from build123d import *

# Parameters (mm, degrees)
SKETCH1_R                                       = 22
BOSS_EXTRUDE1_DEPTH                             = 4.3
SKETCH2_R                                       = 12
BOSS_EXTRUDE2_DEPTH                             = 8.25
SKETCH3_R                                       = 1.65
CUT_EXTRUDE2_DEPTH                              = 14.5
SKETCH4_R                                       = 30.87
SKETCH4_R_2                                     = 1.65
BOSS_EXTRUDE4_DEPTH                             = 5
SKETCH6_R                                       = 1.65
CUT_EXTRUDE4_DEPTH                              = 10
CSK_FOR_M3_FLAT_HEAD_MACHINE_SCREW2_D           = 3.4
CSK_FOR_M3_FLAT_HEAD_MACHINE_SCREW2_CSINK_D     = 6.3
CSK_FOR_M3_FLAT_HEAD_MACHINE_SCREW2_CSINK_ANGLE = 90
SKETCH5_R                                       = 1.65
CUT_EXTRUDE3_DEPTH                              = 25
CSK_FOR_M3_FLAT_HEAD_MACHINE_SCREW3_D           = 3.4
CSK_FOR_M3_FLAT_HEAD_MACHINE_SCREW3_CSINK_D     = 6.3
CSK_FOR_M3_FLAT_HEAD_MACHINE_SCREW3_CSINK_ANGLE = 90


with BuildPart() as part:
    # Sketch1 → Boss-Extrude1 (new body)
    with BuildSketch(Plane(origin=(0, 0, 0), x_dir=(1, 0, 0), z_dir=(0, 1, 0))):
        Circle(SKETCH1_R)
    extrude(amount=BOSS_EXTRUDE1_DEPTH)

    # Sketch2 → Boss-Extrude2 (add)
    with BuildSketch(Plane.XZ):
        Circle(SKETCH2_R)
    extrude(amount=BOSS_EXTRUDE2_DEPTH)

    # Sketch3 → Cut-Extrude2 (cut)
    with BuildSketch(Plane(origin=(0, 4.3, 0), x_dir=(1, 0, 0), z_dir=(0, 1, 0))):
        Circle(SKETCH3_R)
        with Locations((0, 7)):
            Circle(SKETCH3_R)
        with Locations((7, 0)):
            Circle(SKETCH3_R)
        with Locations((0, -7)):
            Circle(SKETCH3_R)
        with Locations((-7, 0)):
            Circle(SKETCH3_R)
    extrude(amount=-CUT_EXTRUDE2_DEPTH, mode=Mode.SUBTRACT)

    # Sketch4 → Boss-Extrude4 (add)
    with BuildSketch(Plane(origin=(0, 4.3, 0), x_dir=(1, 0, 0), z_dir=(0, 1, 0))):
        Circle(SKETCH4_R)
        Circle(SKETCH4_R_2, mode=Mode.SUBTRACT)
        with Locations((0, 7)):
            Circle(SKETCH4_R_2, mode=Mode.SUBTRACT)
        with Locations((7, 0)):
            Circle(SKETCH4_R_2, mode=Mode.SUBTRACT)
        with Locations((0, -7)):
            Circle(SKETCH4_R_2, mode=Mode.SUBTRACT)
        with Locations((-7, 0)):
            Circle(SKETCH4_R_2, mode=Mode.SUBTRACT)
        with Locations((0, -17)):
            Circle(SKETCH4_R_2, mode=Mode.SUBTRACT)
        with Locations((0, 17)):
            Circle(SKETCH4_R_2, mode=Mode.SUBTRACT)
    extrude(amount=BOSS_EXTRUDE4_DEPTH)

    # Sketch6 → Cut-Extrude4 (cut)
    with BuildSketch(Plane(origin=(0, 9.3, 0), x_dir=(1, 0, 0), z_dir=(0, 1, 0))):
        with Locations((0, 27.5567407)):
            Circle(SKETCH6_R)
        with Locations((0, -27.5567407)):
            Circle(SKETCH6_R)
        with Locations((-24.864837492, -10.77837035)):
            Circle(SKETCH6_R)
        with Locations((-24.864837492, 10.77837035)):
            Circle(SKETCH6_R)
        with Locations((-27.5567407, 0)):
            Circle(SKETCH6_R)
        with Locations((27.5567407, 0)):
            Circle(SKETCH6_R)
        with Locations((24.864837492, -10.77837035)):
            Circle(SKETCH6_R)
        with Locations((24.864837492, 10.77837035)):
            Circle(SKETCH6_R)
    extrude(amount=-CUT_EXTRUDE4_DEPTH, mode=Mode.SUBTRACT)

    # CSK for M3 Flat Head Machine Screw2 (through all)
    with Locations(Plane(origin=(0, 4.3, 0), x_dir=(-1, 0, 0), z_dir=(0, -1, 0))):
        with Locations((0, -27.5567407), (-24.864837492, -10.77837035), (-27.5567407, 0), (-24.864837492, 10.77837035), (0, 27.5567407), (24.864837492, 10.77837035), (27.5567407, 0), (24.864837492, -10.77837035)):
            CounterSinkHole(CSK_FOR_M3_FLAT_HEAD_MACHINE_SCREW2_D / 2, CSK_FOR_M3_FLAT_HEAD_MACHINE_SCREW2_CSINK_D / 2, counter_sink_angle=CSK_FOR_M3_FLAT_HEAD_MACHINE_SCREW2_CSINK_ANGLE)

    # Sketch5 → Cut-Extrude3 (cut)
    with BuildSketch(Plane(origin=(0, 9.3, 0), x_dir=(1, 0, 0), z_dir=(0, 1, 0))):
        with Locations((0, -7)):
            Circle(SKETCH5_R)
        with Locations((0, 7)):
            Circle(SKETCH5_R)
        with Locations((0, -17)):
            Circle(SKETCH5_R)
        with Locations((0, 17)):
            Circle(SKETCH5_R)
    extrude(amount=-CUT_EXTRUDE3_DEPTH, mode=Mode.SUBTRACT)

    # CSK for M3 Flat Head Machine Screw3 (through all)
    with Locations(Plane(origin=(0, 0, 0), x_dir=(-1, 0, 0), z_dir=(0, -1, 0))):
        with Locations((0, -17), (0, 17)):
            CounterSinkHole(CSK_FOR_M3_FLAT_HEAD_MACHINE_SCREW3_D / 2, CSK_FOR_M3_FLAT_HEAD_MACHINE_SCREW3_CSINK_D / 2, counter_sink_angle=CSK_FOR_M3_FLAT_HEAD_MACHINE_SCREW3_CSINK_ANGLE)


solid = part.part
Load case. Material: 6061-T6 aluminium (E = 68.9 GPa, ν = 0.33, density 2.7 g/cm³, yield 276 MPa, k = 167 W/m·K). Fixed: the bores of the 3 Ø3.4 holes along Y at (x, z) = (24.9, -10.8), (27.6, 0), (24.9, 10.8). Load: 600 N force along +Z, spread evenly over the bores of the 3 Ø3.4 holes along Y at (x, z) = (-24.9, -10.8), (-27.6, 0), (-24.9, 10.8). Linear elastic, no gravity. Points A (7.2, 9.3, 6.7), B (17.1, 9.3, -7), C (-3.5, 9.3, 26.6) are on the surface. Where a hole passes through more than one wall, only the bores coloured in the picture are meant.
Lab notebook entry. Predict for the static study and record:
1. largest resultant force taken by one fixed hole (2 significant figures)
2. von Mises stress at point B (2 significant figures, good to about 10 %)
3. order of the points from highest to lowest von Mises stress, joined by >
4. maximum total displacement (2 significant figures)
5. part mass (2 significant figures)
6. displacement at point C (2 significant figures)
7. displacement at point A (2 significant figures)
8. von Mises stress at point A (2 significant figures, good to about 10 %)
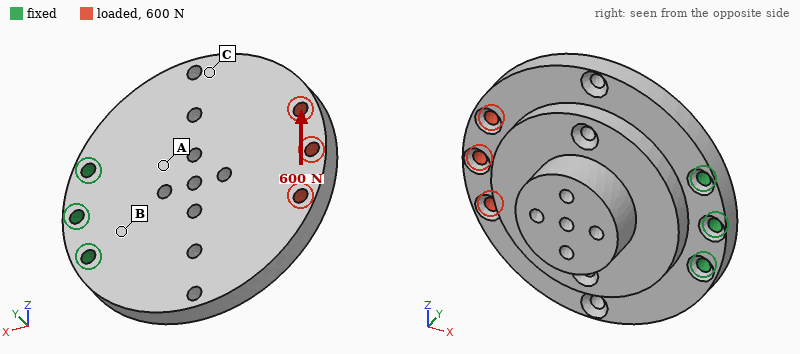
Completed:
1.3 kN
22 MPa
B > A > C
32 µm
64 g
24 µm
10 µm
13 MPa
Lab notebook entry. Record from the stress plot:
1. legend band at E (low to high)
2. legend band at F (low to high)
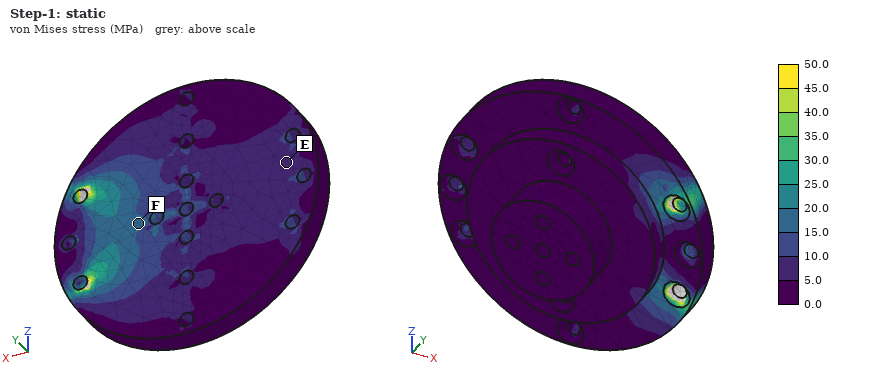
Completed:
5.0 to 10.0 MPa
15.0 to 20.0 MPa
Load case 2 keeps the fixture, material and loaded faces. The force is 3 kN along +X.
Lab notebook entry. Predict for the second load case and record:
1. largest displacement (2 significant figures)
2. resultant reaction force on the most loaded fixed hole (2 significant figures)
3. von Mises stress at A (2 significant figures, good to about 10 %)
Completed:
83 µm
1.2 kN
20 MPa
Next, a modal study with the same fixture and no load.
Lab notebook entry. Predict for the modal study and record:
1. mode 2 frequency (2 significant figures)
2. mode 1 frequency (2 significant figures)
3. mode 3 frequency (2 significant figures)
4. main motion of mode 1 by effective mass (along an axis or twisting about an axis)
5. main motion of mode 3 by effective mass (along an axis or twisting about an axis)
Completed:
4400 Hz
1300 Hz
5500 Hz
along Y
along Z
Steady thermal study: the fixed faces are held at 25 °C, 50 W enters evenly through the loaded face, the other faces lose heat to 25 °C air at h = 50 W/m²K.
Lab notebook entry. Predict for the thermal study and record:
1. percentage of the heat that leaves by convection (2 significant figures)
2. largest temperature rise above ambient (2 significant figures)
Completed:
19 %
53 K
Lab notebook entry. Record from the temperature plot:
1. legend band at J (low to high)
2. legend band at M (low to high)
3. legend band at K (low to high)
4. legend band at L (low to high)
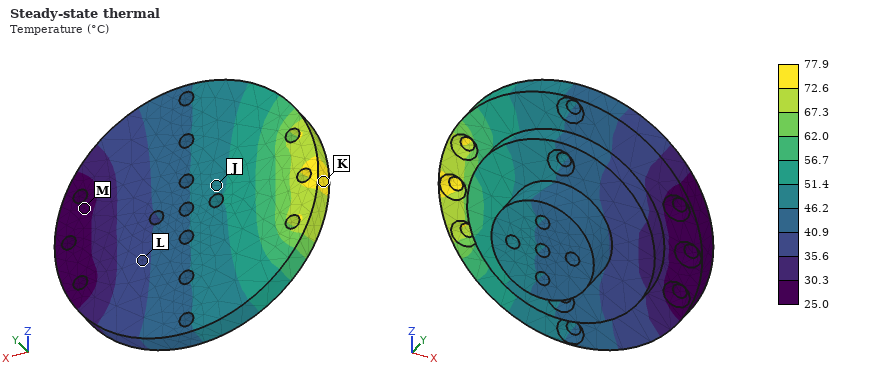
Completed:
46.2 to 51.4 °C
25.0 to 30.3 °C
72.6 to 77.9 °C
35.6 to 40.9 °C
